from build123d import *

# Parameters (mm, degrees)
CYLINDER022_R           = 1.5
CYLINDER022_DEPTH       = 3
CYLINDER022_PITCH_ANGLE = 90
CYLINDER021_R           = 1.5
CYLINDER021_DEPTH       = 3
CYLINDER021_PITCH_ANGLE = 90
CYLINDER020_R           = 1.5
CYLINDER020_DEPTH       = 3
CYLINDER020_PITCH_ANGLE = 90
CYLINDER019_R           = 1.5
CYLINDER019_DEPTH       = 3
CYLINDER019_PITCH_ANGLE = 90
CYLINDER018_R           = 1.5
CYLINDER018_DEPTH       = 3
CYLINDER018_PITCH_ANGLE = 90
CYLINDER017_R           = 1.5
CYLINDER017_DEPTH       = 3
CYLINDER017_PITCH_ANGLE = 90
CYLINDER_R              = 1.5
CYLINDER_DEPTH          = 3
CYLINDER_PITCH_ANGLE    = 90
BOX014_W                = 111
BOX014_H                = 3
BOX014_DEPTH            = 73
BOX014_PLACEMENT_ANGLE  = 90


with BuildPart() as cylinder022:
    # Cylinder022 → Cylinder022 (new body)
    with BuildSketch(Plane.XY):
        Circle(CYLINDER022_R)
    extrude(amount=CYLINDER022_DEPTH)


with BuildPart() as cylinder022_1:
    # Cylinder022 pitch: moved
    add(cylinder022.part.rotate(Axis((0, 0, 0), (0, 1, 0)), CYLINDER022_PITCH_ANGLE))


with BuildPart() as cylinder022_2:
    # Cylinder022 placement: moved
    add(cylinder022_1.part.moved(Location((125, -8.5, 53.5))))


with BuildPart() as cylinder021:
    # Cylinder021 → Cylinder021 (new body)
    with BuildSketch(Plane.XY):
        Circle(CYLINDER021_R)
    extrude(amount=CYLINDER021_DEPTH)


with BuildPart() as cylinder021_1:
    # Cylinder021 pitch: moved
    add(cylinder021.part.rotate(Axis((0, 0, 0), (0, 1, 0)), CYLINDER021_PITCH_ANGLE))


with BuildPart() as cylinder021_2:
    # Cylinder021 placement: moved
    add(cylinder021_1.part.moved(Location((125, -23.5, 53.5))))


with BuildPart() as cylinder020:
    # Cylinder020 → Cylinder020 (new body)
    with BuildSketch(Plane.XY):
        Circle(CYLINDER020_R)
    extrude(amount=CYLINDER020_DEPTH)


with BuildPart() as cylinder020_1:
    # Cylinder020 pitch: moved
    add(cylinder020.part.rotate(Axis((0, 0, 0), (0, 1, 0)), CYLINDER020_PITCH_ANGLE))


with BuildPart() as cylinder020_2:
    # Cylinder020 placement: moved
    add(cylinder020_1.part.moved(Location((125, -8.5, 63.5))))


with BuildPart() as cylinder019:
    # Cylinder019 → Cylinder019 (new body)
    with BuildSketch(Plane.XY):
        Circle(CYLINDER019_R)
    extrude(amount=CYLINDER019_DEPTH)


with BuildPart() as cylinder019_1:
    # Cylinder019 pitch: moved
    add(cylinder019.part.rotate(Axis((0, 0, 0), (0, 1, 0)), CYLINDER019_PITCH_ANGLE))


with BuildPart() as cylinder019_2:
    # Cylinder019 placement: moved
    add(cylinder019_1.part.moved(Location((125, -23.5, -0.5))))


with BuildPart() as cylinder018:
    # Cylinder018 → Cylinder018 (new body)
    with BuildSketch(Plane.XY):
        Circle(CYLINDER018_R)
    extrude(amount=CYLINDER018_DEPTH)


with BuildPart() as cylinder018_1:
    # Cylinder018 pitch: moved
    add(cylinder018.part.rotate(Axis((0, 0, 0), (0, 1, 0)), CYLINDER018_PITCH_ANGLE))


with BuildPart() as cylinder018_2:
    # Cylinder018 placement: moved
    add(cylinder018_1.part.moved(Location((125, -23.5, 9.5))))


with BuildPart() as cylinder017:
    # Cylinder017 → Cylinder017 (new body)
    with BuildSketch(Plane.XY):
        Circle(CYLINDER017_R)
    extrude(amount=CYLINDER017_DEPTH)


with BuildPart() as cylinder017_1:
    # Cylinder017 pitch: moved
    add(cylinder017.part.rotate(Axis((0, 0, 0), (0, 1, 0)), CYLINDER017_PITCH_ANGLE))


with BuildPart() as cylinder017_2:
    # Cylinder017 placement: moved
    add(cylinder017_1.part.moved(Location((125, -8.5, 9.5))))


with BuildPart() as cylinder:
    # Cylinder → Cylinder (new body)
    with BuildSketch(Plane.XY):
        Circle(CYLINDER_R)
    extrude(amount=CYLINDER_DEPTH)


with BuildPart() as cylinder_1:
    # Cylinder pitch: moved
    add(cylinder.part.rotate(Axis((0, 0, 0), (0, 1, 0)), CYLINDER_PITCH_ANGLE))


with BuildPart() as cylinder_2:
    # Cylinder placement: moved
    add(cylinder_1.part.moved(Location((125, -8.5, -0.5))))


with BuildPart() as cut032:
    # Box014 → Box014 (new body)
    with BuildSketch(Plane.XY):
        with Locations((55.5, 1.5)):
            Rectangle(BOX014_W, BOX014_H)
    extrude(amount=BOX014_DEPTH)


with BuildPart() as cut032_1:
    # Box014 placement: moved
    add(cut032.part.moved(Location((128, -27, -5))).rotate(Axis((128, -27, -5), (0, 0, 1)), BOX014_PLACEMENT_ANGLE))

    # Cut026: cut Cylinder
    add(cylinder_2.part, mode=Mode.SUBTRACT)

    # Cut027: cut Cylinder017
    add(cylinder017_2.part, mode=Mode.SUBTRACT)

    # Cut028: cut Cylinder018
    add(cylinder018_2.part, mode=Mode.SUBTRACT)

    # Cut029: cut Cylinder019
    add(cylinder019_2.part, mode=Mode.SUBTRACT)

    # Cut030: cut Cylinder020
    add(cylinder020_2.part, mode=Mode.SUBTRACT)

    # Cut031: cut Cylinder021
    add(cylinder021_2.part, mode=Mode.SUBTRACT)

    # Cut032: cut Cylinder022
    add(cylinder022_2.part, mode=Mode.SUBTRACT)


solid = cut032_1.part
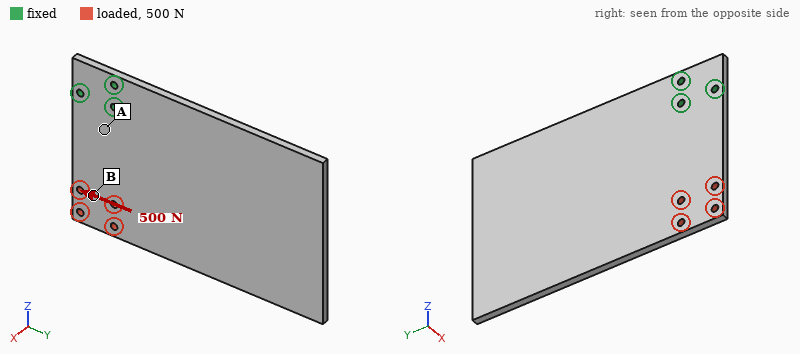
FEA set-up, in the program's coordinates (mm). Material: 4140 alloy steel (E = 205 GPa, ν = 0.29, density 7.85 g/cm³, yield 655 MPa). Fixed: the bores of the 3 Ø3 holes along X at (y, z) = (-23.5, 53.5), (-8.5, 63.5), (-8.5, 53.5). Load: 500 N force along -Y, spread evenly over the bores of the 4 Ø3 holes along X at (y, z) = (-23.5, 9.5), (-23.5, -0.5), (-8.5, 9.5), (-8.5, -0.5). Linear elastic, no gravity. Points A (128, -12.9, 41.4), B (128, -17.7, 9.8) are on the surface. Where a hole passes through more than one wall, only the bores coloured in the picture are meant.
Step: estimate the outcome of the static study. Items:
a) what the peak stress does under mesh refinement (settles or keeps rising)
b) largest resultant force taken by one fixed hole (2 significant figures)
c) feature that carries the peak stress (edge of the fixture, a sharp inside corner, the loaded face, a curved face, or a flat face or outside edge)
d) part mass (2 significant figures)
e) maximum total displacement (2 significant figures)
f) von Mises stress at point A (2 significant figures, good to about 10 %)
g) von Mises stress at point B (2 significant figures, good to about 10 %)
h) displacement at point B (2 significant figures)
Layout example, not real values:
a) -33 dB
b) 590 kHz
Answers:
a) keeps rising
b) 1.1 kN
c) edge of the fixture
d) 190 g
e) 30 µm
f) 19 MPa
g) 5.9 MPa
h) 13 µm
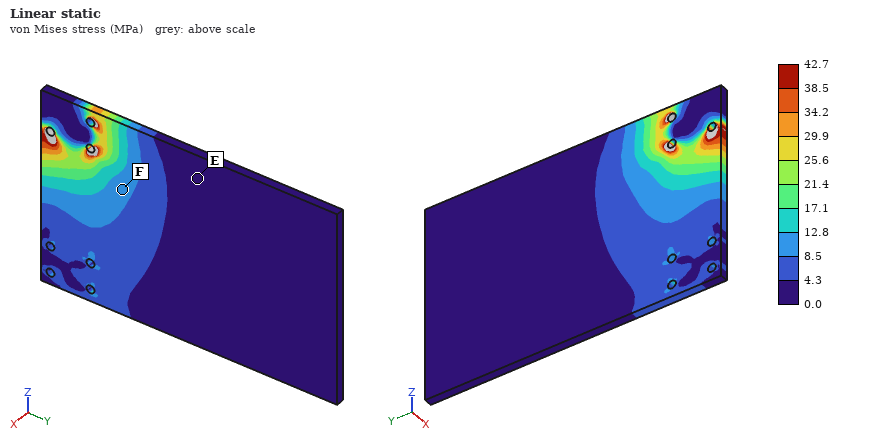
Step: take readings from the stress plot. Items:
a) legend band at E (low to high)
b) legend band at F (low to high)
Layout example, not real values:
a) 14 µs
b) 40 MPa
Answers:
a) 0.0 to 4.3 MPa
b) 8.5 to 12.8 MPa
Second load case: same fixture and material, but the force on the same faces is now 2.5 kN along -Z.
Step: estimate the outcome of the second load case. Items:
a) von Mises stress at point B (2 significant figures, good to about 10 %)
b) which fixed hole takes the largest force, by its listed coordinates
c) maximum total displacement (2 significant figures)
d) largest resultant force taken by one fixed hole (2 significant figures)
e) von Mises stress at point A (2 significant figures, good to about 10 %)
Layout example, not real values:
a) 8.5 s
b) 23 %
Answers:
a) 25 MPa
b) (-23.5, 53.5)
c) 13 µm
d) 1.2 kN
e) 27 MPa
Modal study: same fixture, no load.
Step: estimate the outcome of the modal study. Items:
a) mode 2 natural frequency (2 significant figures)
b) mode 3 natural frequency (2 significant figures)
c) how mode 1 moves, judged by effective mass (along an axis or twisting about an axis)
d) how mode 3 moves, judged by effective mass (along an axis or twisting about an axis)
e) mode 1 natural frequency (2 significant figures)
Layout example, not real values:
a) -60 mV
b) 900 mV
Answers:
a) 520 Hz
b) 1100 Hz
c) along X
d) along X
e) 230 Hz
